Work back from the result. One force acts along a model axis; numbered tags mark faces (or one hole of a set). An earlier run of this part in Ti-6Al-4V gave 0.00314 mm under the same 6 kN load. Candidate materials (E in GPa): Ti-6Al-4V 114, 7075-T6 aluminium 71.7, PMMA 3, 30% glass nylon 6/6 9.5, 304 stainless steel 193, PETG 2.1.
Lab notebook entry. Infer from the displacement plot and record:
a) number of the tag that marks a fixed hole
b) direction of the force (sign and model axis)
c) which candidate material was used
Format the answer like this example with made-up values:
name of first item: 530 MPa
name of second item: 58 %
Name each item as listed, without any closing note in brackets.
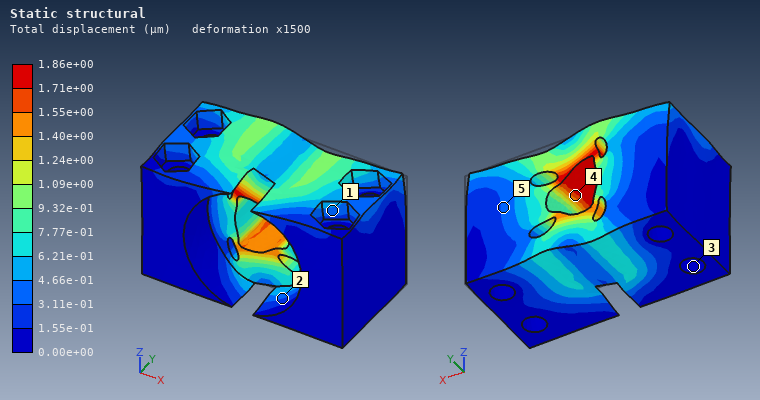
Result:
number of the tag that marks a fixed hole: 3
direction of the force: -X
which candidate material was used: 304 stainless steel
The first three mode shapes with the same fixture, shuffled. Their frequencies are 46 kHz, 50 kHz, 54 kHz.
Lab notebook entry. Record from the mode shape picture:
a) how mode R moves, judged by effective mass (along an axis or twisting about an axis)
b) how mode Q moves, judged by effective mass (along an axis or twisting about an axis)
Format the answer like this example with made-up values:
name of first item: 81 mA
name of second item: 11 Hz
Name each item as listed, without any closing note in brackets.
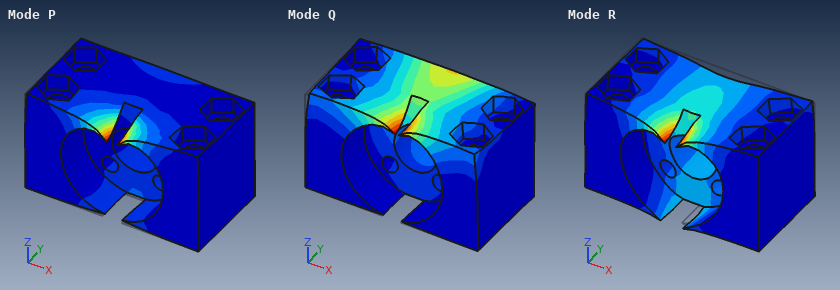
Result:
how mode R moves, judged by effective mass: along Z
how mode Q moves, judged by effective mass: along Y
